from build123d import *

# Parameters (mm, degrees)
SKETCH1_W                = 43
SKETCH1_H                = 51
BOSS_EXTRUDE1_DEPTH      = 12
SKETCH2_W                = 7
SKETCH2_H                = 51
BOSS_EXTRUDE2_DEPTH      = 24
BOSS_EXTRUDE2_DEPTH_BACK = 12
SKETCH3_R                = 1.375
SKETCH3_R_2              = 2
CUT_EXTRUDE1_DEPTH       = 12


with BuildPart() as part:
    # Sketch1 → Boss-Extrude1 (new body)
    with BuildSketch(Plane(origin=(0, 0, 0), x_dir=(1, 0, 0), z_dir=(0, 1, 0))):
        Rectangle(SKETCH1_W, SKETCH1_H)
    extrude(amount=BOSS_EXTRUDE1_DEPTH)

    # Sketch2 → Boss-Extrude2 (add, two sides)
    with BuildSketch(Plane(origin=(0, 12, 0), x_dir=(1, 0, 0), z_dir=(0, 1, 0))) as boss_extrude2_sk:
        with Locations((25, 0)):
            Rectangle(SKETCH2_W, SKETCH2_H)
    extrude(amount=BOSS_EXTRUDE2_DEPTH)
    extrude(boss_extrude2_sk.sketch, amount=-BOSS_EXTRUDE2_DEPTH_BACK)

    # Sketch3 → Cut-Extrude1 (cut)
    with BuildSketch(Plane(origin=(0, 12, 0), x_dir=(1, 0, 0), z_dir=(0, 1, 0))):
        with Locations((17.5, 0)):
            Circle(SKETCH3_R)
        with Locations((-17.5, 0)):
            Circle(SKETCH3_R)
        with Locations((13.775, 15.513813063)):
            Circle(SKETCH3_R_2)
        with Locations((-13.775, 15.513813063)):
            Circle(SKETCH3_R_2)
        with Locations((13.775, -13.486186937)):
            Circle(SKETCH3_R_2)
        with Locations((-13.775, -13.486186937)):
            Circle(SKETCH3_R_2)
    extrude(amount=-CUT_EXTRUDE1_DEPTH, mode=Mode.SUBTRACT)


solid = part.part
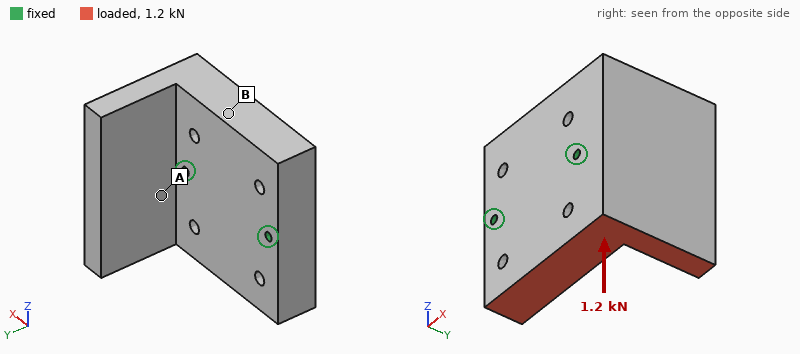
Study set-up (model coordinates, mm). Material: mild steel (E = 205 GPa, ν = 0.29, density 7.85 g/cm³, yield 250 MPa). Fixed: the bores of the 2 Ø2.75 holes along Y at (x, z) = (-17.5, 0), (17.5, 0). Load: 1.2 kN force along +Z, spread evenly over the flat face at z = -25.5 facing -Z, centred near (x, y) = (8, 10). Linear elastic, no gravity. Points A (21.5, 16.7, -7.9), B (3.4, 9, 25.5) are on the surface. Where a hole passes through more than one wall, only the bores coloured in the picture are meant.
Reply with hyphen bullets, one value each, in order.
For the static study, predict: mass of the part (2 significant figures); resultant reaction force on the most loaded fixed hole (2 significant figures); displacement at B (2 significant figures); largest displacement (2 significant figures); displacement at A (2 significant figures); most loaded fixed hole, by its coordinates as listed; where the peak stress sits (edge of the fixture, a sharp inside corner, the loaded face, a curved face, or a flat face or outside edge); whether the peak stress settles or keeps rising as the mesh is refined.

- 300 g
- 870 N
- 0.85 µm
- 2.6 µm
- 0.95 µm
- (17.5, 0)
- edge of the fixture
- keeps rising
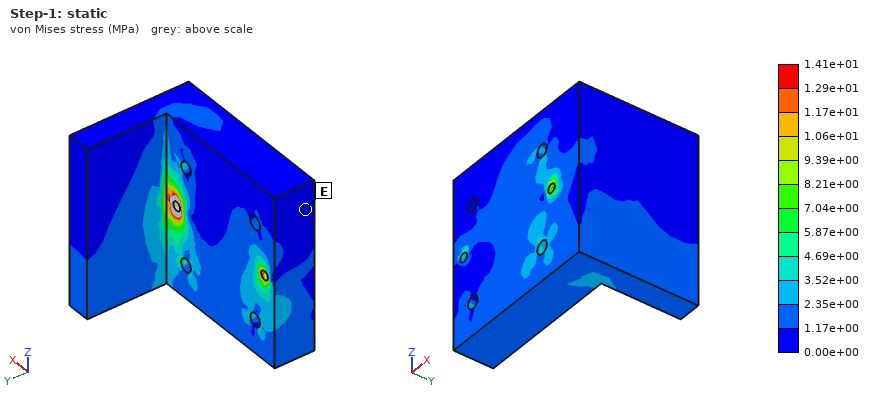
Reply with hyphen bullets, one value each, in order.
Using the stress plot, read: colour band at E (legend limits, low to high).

- 0.00e+00 to 1.17e+00 MPa
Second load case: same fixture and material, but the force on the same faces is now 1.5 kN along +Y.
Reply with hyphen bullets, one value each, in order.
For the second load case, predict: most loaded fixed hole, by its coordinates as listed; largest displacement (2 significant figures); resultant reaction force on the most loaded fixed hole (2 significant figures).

- (17.5, 0)
- 13 µm
- 1.0 kN
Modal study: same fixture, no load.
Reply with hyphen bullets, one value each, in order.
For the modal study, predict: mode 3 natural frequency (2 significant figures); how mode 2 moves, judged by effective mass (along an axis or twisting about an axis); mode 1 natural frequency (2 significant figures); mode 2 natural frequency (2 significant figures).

- 9600 Hz
- along X
- 5800 Hz
- 6100 Hz
